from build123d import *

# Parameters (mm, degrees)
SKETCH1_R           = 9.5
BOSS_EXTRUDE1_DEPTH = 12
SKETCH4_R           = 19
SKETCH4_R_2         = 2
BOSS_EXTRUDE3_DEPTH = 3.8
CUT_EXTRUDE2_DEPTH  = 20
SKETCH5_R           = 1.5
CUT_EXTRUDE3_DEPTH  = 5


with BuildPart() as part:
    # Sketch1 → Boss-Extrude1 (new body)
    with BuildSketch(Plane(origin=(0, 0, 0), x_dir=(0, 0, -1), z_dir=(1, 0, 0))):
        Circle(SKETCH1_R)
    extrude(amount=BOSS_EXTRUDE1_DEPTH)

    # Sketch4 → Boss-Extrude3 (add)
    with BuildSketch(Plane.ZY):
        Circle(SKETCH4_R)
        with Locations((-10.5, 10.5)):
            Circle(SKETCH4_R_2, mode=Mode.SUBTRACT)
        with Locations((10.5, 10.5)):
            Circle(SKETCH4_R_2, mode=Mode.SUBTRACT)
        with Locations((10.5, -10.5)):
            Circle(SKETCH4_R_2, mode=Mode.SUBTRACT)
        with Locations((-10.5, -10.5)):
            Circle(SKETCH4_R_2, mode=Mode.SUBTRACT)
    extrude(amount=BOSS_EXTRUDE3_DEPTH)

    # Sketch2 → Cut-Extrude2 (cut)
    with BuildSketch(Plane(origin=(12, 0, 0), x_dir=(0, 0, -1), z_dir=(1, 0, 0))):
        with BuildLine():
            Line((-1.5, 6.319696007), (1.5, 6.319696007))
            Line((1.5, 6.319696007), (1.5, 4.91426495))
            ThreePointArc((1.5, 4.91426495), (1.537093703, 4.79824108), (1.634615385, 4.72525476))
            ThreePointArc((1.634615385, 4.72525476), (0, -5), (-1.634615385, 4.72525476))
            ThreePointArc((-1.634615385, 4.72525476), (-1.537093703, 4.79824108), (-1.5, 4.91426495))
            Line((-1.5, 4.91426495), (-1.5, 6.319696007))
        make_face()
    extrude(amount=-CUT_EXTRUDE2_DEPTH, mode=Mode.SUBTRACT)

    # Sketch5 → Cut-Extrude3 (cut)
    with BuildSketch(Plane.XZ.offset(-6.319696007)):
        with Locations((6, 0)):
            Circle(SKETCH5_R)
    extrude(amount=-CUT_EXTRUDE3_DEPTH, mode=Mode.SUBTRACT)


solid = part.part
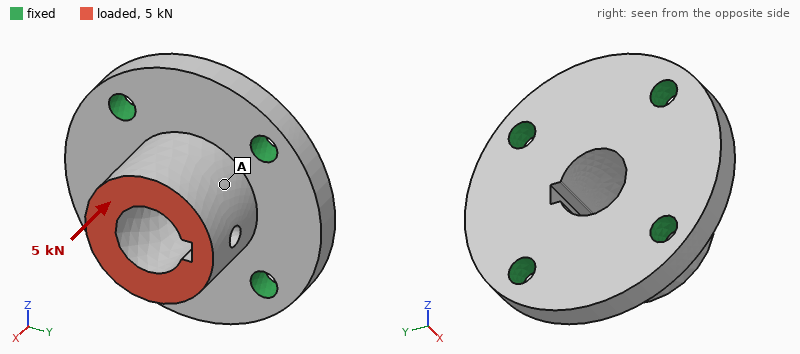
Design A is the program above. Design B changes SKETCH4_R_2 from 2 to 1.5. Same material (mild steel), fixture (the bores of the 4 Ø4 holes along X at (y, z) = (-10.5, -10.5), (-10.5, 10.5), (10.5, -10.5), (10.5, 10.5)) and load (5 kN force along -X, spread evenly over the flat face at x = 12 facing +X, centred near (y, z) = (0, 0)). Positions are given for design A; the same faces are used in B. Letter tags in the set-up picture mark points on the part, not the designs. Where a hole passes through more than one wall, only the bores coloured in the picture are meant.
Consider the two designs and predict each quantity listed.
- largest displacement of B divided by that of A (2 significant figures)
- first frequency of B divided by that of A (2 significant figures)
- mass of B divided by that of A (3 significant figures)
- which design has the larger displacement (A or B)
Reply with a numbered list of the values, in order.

1. 1.2
2. 0.93
3. 1.01
4. B
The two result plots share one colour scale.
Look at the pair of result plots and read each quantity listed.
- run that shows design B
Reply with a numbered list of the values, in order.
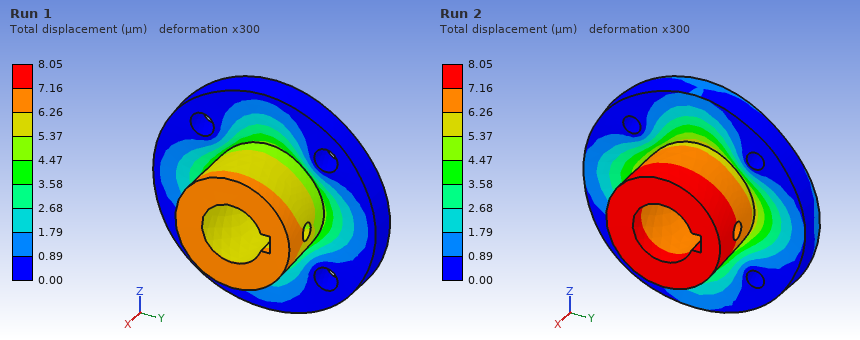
1. Run 2
